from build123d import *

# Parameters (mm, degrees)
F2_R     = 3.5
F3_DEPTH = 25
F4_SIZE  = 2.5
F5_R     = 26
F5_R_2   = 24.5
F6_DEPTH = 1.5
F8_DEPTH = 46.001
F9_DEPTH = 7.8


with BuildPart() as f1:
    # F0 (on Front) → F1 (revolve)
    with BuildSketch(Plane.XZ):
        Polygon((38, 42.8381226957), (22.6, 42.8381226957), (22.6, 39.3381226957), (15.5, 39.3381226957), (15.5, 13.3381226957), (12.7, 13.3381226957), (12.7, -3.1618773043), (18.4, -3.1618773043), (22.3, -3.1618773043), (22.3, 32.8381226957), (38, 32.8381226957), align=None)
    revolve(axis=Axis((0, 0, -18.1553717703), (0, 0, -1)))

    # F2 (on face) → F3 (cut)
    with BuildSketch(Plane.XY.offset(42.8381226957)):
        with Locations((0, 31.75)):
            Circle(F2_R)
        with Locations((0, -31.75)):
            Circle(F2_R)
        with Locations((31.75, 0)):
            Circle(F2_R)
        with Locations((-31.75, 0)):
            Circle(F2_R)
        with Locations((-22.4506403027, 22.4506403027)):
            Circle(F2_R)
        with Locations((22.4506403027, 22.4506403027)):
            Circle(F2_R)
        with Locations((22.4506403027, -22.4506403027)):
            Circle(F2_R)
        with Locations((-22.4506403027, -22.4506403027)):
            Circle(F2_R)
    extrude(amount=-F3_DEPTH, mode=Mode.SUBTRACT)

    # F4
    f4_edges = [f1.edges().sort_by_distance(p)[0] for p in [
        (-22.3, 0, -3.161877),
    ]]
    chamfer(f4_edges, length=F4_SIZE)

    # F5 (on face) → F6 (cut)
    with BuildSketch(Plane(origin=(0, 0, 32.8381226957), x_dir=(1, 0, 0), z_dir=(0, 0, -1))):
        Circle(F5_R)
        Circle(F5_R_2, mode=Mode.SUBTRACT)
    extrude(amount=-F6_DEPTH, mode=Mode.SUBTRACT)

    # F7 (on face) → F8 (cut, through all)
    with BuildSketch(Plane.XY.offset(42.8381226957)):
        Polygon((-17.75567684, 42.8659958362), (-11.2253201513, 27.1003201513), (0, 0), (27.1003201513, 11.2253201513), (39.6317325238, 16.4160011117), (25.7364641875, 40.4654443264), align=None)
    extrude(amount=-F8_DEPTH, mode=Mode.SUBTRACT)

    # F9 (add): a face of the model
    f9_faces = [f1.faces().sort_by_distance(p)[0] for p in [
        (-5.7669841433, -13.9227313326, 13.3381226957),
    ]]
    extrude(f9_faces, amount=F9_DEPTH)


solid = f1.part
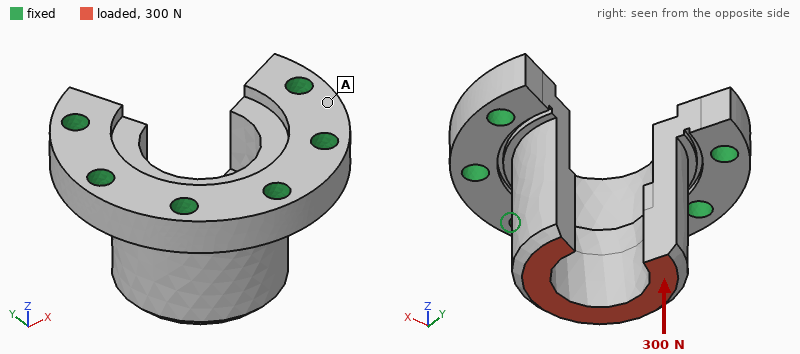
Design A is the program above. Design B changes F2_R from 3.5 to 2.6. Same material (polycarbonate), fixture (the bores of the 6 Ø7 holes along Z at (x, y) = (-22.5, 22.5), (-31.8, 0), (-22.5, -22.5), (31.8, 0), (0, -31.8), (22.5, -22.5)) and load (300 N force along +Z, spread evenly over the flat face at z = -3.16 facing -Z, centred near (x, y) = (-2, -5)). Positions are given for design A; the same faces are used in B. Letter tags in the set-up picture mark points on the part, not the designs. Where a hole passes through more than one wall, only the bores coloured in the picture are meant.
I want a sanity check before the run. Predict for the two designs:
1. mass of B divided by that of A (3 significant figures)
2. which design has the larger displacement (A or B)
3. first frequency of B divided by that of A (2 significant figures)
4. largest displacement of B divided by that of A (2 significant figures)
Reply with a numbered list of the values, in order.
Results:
1. 1.02
2. B
3. 0.98
4. 1.1
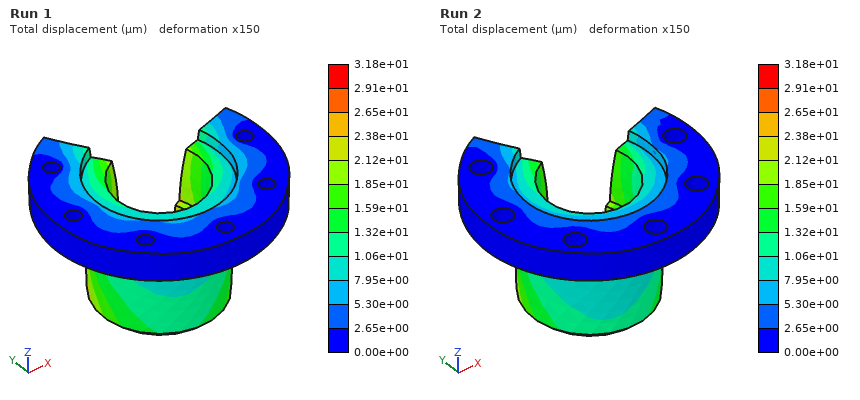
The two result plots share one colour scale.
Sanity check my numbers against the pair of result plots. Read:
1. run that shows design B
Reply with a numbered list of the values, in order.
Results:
1. Run 1
